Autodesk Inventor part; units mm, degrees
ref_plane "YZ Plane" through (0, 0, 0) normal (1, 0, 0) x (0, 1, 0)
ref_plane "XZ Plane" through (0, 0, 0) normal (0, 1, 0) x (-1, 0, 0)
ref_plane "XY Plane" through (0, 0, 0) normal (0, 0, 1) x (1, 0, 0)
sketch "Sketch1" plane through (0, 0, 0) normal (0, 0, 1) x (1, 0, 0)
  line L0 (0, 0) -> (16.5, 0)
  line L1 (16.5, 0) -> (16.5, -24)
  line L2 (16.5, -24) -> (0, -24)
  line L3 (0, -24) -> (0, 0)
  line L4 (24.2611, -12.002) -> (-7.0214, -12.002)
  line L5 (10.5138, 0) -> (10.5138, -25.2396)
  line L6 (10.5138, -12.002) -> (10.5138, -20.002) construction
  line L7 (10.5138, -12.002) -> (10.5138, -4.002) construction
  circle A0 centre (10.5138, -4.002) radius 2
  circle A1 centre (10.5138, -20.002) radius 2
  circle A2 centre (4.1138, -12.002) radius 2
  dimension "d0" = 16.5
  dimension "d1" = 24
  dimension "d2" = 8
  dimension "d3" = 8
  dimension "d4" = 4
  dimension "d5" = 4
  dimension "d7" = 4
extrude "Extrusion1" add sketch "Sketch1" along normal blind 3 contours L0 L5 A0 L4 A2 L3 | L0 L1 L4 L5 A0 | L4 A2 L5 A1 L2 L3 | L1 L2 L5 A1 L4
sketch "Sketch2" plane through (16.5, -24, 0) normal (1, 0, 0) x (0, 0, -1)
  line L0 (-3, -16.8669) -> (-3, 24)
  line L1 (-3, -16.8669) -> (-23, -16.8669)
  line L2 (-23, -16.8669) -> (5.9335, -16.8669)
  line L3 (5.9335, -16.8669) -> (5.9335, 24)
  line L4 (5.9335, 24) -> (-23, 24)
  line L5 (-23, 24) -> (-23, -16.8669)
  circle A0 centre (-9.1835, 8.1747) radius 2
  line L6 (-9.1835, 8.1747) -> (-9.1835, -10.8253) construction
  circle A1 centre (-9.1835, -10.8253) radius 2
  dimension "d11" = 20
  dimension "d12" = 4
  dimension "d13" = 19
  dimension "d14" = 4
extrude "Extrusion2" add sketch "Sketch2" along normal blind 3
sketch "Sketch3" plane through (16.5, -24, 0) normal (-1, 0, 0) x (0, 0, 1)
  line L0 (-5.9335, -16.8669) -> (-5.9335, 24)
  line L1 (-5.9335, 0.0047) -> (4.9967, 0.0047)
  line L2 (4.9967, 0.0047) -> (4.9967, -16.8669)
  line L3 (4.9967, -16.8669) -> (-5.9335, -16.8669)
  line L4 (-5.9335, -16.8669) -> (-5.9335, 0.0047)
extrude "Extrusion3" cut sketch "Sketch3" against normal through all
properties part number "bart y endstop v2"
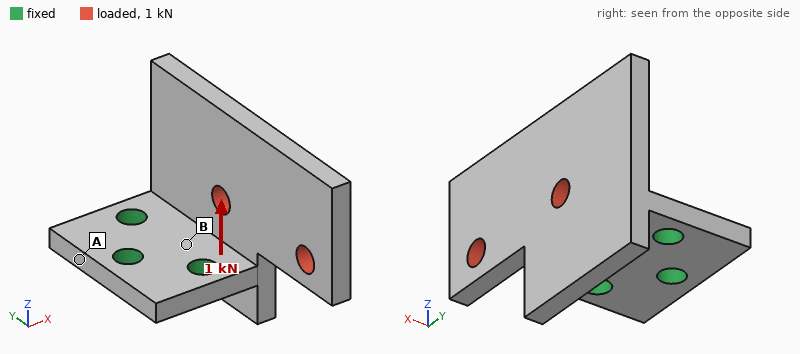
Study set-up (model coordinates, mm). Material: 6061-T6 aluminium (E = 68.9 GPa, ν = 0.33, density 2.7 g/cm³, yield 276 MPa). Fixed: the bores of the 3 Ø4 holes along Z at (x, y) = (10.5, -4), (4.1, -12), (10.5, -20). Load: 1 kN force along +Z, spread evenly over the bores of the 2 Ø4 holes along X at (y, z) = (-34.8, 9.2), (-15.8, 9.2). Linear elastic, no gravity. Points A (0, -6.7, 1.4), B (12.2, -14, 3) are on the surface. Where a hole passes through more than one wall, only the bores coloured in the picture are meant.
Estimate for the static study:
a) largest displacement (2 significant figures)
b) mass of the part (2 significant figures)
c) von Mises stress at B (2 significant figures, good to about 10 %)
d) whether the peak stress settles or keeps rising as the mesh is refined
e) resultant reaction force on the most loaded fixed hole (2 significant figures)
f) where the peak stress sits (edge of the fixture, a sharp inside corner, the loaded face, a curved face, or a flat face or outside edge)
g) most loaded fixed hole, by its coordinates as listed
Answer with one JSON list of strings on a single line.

["0.26 mm", "11 g", "86 MPa", "keeps rising", "1.3 kN", "edge of the fixture", "(10.5, -20)"]
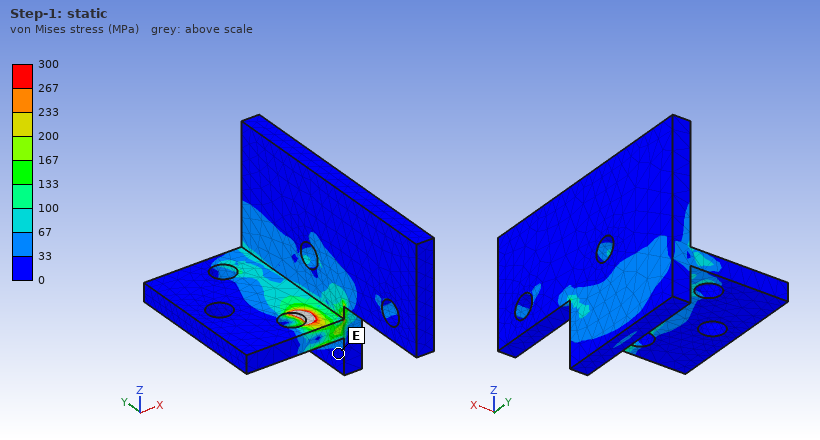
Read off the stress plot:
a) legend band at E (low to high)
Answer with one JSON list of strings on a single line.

["0 to 33 MPa"]
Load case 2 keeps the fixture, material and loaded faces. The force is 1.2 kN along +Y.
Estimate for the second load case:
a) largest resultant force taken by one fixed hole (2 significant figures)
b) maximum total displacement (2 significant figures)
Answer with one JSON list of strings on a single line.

["910 N", "90 µm"]
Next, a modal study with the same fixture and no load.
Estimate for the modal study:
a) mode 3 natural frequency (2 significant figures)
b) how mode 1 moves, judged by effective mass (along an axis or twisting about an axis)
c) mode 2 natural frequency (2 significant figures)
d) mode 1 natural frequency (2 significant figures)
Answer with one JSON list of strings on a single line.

["6400 Hz", "along X", "4500 Hz", "2500 Hz"]
